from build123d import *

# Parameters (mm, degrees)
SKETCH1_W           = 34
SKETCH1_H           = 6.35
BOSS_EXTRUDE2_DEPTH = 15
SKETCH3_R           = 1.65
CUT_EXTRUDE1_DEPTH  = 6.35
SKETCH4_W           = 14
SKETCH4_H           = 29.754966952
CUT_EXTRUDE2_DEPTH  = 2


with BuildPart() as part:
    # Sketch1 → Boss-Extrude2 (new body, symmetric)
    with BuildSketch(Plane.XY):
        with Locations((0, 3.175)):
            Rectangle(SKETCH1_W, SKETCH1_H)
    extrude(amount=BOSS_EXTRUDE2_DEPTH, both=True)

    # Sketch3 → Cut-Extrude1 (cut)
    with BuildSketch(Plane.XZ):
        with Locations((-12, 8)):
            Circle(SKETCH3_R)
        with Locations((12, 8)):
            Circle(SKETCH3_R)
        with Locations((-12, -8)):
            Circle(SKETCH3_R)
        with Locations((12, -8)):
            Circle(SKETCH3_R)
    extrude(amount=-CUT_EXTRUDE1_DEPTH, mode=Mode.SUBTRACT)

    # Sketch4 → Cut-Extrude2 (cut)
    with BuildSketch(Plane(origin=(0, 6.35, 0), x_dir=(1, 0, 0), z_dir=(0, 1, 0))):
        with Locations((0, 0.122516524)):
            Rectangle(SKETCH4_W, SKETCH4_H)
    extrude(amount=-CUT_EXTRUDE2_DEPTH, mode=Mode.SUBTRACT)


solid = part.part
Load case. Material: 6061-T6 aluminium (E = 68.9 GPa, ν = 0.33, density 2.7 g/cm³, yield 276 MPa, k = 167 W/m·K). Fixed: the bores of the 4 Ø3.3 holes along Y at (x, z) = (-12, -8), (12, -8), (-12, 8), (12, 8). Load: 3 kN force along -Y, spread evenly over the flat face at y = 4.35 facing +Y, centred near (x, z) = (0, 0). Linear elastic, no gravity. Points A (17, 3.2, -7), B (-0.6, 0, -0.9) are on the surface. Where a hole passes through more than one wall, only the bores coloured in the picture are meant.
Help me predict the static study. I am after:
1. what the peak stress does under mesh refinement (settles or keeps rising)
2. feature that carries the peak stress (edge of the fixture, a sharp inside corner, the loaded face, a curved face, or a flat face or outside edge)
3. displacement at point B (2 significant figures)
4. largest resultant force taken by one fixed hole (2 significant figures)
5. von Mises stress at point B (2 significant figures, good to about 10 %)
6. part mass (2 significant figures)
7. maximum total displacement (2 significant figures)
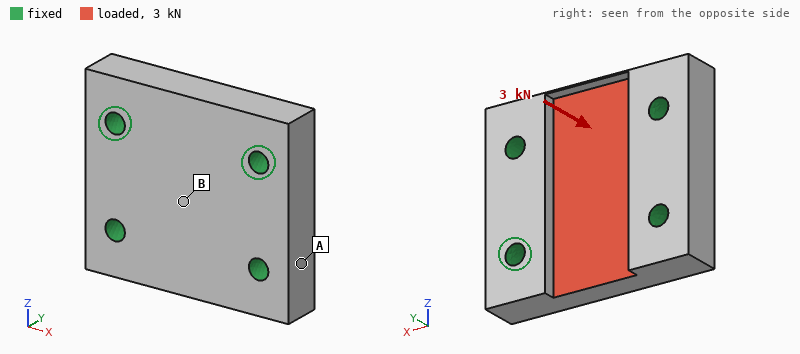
keeps rising
edge of the fixture
10 µm
780 N
35 MPa
15 g
12 µm
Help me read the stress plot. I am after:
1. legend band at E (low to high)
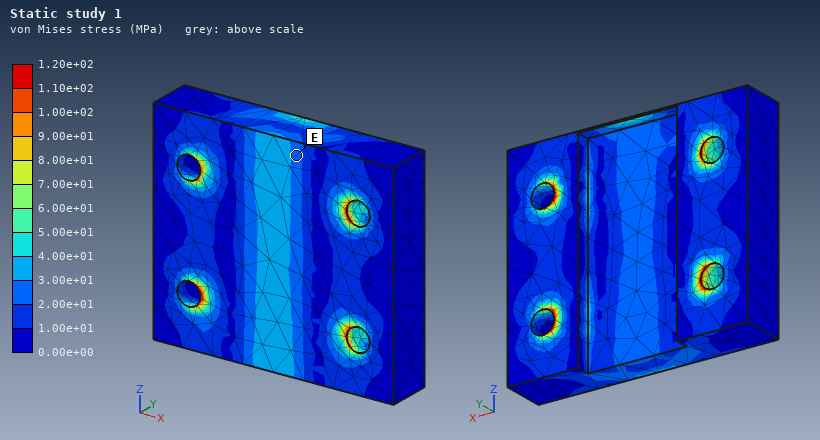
2.00e+01 to 3.00e+01 MPa
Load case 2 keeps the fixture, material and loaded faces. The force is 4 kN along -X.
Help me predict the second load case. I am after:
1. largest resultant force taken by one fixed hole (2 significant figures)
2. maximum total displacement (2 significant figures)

1.0 kN
3.3 µm
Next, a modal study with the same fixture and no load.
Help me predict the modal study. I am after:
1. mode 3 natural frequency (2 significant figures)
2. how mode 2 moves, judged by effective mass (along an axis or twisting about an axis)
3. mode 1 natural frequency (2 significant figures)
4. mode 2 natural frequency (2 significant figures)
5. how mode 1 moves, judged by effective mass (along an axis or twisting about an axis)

52 kHz
twisting about X
40 kHz
43 kHz
along Y
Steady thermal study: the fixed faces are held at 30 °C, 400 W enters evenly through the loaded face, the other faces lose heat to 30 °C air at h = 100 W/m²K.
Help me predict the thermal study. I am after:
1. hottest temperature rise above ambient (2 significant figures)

80 K
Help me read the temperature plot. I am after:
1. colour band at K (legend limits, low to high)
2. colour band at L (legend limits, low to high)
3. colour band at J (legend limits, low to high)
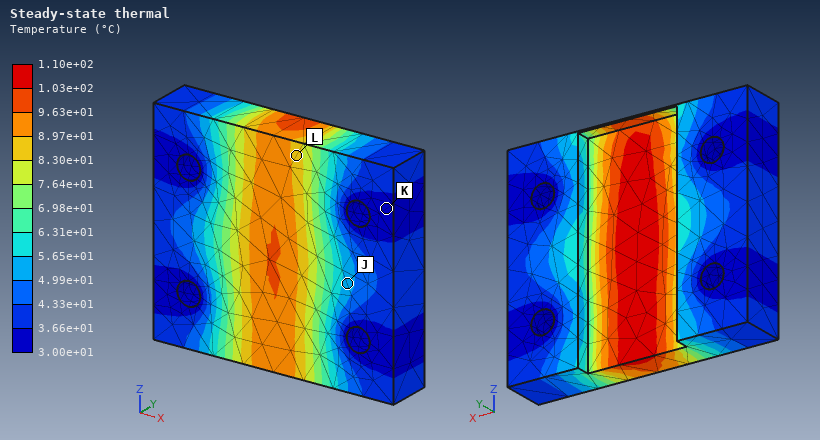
3.00e+01 to 3.66e+01 °C
8.30e+01 to 8.97e+01 °C
4.99e+01 to 5.65e+01 °C
